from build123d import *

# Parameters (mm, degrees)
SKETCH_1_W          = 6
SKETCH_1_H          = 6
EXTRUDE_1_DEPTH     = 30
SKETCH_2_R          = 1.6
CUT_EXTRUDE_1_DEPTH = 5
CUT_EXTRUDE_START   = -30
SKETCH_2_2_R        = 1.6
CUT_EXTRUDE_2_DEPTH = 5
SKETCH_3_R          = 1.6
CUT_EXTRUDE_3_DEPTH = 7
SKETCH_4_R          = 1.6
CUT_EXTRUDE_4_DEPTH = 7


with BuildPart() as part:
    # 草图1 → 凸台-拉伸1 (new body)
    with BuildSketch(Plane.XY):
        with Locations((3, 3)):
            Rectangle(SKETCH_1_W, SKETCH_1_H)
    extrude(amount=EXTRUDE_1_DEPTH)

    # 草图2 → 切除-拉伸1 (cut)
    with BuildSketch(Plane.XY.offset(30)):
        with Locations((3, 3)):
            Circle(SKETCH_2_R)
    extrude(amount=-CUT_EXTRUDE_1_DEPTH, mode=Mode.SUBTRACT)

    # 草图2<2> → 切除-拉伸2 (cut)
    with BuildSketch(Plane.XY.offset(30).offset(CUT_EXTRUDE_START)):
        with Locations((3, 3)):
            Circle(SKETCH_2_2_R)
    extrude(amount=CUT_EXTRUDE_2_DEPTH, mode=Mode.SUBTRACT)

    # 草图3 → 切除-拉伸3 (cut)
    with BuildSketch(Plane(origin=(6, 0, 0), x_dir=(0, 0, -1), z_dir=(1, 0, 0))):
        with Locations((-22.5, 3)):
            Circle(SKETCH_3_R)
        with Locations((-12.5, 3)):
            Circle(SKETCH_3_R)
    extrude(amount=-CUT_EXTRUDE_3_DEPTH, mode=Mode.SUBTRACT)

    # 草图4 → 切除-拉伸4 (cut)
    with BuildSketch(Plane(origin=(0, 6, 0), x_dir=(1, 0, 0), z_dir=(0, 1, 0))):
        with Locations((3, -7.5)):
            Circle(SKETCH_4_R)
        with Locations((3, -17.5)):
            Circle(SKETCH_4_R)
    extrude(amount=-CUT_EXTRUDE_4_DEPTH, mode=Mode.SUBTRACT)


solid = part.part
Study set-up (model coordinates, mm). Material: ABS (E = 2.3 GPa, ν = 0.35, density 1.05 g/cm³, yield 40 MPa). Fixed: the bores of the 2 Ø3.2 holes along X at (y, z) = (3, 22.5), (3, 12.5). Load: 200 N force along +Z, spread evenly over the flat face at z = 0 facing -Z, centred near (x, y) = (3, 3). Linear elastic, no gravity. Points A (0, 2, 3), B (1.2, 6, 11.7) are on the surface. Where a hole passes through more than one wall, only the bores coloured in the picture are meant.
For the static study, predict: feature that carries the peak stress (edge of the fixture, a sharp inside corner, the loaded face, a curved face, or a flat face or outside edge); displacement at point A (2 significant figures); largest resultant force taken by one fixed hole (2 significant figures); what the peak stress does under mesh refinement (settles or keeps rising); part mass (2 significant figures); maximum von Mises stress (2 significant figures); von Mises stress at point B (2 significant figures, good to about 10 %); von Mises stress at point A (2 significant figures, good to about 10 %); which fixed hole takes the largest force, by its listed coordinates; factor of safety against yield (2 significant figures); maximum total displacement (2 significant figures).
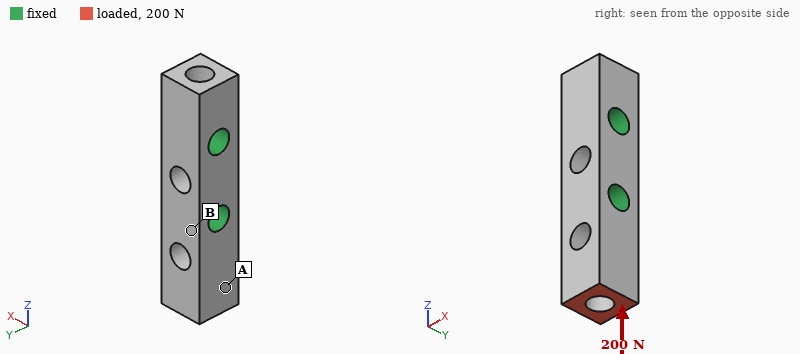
a curved face
34 µm
200 N
settles
0.85 g
24 MPa
3.8 MPa
8.5 MPa
(3, 12.5)
1.7
45 µm
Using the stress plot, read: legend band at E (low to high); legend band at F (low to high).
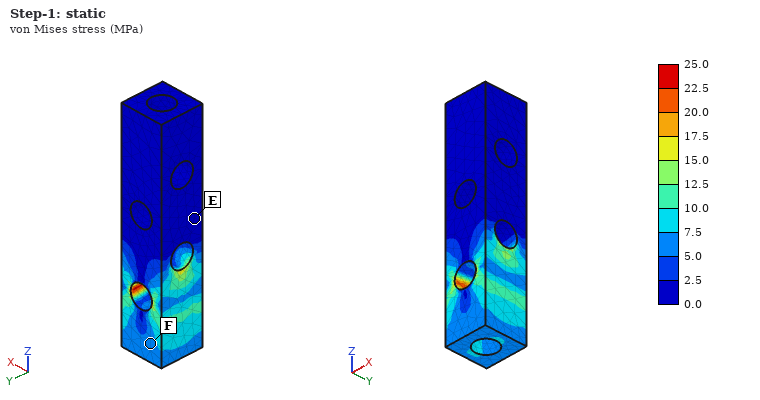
0.0 to 2.5 MPa
5.0 to 7.5 MPa
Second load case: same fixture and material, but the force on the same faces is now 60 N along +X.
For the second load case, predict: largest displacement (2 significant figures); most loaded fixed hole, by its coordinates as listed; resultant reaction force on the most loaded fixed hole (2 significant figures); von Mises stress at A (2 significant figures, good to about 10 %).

0.22 mm
(3, 12.5)
61 N
5.2 MPa
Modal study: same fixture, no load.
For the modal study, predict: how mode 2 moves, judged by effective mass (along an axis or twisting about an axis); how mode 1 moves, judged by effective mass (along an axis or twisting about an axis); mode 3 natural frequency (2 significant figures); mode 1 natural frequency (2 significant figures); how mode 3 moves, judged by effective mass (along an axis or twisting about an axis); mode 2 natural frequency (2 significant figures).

along X
along Y
15 kHz
7600 Hz
twisting about Z
8300 Hz
